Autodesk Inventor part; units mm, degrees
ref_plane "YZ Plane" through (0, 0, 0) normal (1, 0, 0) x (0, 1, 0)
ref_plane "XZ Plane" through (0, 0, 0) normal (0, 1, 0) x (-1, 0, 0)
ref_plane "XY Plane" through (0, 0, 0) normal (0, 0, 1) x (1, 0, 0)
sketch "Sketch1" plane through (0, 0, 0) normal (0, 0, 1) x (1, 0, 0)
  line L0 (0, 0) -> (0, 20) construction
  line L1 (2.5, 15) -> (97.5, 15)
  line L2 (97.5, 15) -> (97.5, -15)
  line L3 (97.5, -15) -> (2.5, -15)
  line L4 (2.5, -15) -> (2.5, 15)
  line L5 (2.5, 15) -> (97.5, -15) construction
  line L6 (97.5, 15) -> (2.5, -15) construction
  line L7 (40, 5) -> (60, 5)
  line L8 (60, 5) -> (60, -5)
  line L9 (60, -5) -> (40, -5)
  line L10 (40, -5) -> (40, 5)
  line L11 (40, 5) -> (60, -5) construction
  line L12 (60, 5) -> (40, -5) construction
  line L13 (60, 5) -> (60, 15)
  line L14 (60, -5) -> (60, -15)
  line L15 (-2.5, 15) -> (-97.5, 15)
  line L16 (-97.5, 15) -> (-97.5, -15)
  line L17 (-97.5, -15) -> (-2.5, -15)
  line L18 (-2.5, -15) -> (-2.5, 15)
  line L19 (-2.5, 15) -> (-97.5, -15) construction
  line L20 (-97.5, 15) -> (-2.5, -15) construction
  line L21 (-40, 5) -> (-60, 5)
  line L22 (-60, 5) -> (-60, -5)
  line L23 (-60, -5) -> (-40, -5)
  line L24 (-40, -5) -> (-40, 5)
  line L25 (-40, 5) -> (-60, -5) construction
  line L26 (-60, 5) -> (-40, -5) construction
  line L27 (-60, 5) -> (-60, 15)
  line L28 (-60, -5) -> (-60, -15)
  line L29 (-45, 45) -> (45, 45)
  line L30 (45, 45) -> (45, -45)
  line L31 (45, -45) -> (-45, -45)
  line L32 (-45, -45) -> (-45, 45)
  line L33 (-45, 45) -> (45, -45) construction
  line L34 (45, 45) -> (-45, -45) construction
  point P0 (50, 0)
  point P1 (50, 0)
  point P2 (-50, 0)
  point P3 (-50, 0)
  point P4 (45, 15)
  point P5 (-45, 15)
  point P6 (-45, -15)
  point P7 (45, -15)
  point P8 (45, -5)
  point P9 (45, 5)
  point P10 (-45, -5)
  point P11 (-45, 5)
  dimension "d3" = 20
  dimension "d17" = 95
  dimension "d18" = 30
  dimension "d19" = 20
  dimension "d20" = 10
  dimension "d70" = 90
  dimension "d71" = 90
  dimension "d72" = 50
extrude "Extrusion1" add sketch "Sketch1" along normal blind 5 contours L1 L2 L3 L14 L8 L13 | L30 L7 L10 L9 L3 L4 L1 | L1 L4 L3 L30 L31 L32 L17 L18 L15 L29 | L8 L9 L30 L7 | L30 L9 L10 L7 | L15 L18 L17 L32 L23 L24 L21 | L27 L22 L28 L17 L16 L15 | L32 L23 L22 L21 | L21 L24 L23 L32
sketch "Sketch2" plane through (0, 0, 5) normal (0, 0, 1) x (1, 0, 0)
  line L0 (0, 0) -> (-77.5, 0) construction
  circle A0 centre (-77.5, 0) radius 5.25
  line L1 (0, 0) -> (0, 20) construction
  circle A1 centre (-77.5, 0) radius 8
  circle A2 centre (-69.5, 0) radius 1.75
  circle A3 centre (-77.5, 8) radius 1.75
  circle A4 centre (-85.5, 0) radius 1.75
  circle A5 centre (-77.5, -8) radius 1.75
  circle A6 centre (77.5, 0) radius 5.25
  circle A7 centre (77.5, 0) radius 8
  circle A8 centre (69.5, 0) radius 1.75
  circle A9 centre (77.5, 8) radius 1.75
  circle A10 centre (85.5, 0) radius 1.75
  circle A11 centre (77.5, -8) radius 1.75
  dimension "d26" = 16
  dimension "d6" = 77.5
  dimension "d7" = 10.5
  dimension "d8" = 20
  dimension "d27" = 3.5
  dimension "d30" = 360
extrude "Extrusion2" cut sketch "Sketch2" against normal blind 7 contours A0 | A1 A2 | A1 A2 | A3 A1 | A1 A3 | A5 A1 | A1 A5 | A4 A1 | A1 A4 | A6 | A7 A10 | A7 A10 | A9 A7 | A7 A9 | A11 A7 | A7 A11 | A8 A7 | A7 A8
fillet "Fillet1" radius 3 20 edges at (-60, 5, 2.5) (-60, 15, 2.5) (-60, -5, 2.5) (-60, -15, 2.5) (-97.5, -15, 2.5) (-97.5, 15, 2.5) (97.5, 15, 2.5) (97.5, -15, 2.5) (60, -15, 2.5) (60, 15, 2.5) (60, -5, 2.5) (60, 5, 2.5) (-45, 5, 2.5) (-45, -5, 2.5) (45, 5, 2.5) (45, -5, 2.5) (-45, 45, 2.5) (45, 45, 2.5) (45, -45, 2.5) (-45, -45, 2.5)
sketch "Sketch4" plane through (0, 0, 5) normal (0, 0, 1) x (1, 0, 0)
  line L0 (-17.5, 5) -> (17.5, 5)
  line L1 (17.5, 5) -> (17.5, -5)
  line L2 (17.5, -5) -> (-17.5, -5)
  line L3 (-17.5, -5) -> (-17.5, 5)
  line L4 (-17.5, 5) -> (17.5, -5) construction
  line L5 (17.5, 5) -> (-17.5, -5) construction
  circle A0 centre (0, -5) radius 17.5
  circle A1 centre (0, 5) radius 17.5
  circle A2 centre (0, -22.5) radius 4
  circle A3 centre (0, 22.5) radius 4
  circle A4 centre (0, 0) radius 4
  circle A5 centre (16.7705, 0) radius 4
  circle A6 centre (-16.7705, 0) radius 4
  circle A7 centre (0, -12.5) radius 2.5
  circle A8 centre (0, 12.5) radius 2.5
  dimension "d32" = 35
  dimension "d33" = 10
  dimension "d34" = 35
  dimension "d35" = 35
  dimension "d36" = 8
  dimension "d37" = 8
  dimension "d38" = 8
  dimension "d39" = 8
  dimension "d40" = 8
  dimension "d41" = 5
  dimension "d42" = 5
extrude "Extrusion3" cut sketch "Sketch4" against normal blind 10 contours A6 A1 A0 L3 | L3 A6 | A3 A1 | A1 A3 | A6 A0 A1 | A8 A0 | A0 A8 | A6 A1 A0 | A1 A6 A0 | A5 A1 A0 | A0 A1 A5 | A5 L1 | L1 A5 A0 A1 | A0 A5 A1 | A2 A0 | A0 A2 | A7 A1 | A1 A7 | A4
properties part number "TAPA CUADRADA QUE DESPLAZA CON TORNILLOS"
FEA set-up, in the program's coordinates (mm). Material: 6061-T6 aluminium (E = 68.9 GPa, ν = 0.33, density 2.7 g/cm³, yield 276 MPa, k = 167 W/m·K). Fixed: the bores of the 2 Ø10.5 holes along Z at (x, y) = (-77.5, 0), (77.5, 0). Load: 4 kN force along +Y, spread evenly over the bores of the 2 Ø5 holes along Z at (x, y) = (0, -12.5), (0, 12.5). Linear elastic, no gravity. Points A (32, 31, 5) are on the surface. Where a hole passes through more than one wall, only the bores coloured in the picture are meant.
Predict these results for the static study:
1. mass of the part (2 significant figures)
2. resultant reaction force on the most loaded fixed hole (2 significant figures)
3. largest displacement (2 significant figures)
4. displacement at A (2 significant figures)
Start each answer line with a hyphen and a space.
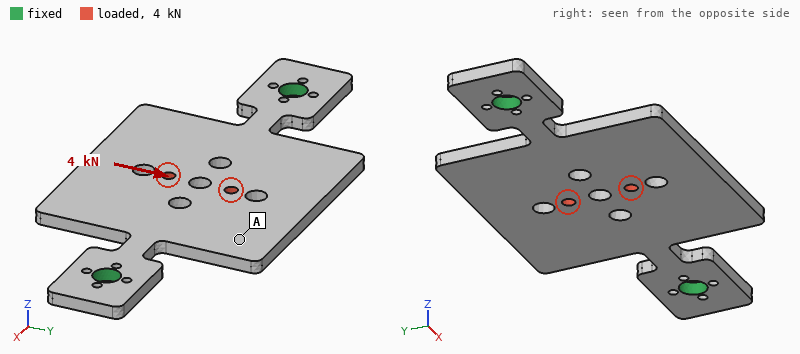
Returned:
- 140 g
- 2.0 kN
- 0.12 mm
- 0.11 mm
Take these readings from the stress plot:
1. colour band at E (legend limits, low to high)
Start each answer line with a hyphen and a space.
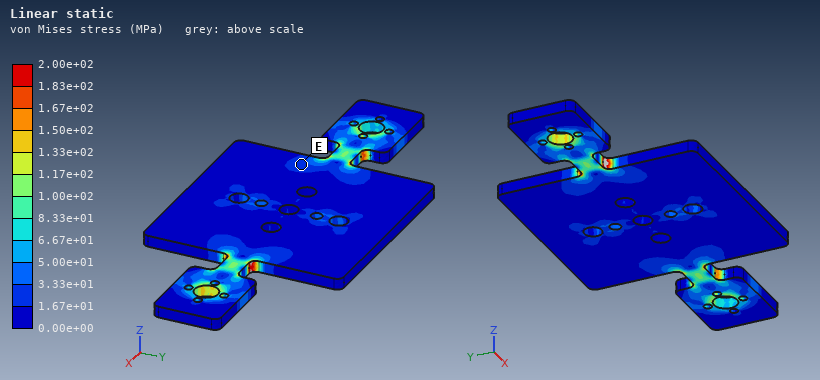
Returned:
- 1.67e+01 to 3.33e+01 MPa
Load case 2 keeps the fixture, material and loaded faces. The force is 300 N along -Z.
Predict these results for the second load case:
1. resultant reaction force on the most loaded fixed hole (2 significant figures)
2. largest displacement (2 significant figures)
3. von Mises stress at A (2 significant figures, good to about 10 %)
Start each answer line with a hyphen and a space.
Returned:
- 150 N
- 0.21 mm
- 7.4 MPa
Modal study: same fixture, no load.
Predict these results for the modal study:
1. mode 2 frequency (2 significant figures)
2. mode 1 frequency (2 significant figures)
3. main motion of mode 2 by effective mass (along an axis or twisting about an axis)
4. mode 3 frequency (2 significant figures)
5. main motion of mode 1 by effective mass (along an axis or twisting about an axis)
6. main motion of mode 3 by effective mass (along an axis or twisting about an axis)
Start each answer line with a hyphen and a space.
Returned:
- 690 Hz
- 460 Hz
- along Z
- 1800 Hz
- twisting about X
- twisting about Y
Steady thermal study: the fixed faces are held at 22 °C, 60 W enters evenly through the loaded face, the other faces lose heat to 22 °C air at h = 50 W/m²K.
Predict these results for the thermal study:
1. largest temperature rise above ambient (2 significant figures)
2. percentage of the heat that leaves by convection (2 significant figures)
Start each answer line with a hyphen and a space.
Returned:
- 58 K
- 64 %
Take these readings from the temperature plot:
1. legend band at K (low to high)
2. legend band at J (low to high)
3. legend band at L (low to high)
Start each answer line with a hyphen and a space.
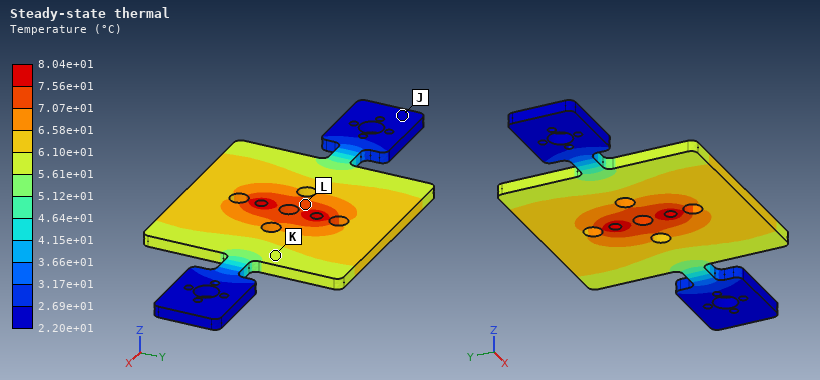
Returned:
- 5.61e+01 to 6.10e+01 °C
- 2.20e+01 to 2.69e+01 °C
- 7.07e+01 to 7.56e+01 °C
